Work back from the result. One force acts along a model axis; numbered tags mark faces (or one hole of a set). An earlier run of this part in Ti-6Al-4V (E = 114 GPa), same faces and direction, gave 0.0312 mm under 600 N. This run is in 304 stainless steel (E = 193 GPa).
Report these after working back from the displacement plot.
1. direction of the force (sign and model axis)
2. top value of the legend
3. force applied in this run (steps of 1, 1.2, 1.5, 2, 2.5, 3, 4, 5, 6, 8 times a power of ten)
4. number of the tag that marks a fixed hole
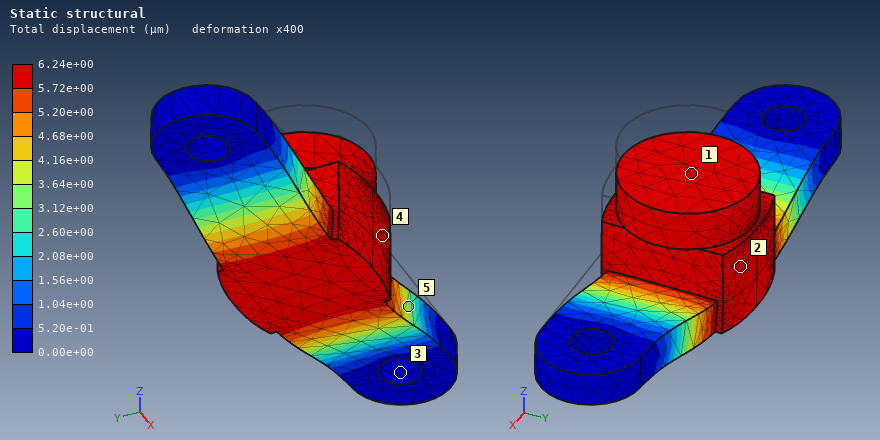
-Z
6.24e+00 µm
200 N
3
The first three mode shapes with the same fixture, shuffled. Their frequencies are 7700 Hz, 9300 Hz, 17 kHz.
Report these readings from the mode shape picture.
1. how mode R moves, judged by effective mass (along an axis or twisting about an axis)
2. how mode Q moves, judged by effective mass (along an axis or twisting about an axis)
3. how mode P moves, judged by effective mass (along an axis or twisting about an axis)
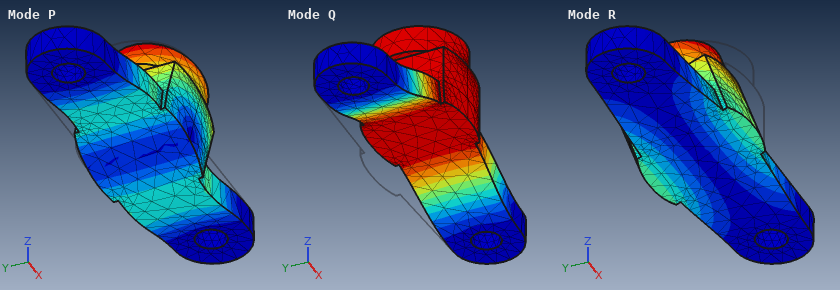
along Y
along Z
along X
